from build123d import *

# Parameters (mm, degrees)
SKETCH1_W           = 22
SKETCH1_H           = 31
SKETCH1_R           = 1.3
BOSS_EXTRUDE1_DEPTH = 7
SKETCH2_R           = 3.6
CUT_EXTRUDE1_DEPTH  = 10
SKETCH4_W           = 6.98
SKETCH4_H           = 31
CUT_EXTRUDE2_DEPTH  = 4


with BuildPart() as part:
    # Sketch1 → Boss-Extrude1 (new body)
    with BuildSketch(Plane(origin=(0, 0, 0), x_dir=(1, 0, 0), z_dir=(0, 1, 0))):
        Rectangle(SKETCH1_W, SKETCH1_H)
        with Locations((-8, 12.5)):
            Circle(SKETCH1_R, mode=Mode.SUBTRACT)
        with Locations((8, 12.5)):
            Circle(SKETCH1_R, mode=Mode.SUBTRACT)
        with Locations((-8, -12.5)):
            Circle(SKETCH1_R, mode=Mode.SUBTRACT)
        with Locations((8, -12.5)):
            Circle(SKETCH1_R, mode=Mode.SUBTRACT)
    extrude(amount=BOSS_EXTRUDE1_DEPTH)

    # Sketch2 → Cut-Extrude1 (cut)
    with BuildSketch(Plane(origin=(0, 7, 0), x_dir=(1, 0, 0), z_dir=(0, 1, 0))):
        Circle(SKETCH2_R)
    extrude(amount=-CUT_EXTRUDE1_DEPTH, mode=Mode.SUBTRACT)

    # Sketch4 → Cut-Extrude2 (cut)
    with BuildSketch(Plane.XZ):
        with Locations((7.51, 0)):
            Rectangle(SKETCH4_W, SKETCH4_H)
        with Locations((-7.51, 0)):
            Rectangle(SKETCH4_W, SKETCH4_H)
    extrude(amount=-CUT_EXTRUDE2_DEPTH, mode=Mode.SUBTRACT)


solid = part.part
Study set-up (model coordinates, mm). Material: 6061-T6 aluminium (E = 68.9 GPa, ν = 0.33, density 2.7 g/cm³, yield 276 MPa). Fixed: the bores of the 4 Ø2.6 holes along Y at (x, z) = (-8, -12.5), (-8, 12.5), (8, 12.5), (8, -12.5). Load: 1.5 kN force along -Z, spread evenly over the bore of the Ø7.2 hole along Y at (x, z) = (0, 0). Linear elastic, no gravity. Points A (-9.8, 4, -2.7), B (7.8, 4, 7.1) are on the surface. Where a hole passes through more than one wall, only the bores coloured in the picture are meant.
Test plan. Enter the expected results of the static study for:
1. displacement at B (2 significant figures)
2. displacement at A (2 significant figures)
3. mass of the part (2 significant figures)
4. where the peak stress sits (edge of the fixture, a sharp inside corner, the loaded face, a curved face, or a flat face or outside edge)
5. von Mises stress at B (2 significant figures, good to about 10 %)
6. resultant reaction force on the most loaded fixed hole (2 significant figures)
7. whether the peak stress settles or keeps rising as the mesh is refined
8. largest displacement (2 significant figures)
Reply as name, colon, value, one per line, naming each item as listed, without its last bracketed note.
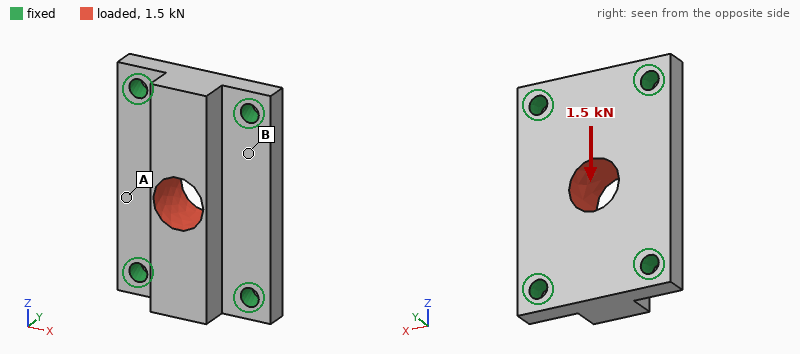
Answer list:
displacement at B: 1.0 µm
displacement at A: 1.1 µm
mass of the part: 7.3 g
where the peak stress sits: edge of the fixture
von Mises stress at B: 14 MPa
resultant reaction force on the most loaded fixed hole: 400 N
whether the peak stress settles or keeps rising as the mesh is refined: keeps rising
largest displacement: 4.3 µm
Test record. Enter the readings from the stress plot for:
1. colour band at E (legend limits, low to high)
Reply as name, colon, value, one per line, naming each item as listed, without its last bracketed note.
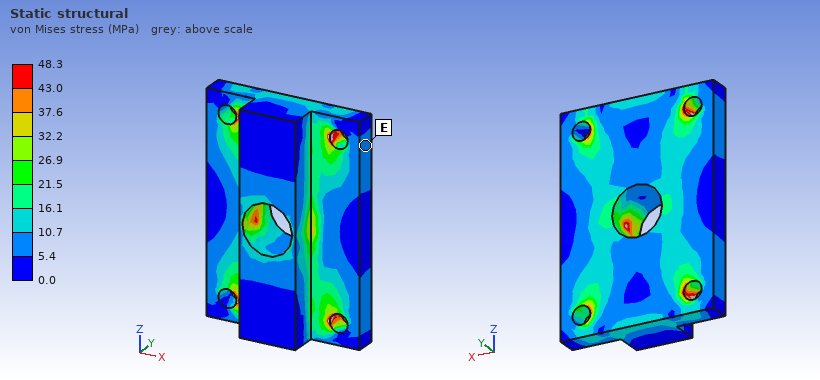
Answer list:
colour band at E: 5.4 to 10.7 MPa
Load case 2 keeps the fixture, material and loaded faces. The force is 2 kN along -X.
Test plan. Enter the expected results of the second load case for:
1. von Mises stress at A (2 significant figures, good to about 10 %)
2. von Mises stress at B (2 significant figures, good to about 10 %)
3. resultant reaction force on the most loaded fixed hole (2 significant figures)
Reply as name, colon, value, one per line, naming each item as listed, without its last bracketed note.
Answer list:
von Mises stress at A: 10 MPa
von Mises stress at B: 26 MPa
resultant reaction force on the most loaded fixed hole: 630 N
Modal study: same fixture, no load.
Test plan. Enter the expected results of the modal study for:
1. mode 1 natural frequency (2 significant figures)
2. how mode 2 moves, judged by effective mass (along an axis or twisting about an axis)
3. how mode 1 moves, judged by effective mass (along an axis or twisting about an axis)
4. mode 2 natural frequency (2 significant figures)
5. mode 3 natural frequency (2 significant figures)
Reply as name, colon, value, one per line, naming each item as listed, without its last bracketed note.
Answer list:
mode 1 natural frequency: 23 kHz
how mode 2 moves, judged by effective mass: twisting about Z
how mode 1 moves, judged by effective mass: along Y
mode 2 natural frequency: 34 kHz
mode 3 natural frequency: 45 kHz
